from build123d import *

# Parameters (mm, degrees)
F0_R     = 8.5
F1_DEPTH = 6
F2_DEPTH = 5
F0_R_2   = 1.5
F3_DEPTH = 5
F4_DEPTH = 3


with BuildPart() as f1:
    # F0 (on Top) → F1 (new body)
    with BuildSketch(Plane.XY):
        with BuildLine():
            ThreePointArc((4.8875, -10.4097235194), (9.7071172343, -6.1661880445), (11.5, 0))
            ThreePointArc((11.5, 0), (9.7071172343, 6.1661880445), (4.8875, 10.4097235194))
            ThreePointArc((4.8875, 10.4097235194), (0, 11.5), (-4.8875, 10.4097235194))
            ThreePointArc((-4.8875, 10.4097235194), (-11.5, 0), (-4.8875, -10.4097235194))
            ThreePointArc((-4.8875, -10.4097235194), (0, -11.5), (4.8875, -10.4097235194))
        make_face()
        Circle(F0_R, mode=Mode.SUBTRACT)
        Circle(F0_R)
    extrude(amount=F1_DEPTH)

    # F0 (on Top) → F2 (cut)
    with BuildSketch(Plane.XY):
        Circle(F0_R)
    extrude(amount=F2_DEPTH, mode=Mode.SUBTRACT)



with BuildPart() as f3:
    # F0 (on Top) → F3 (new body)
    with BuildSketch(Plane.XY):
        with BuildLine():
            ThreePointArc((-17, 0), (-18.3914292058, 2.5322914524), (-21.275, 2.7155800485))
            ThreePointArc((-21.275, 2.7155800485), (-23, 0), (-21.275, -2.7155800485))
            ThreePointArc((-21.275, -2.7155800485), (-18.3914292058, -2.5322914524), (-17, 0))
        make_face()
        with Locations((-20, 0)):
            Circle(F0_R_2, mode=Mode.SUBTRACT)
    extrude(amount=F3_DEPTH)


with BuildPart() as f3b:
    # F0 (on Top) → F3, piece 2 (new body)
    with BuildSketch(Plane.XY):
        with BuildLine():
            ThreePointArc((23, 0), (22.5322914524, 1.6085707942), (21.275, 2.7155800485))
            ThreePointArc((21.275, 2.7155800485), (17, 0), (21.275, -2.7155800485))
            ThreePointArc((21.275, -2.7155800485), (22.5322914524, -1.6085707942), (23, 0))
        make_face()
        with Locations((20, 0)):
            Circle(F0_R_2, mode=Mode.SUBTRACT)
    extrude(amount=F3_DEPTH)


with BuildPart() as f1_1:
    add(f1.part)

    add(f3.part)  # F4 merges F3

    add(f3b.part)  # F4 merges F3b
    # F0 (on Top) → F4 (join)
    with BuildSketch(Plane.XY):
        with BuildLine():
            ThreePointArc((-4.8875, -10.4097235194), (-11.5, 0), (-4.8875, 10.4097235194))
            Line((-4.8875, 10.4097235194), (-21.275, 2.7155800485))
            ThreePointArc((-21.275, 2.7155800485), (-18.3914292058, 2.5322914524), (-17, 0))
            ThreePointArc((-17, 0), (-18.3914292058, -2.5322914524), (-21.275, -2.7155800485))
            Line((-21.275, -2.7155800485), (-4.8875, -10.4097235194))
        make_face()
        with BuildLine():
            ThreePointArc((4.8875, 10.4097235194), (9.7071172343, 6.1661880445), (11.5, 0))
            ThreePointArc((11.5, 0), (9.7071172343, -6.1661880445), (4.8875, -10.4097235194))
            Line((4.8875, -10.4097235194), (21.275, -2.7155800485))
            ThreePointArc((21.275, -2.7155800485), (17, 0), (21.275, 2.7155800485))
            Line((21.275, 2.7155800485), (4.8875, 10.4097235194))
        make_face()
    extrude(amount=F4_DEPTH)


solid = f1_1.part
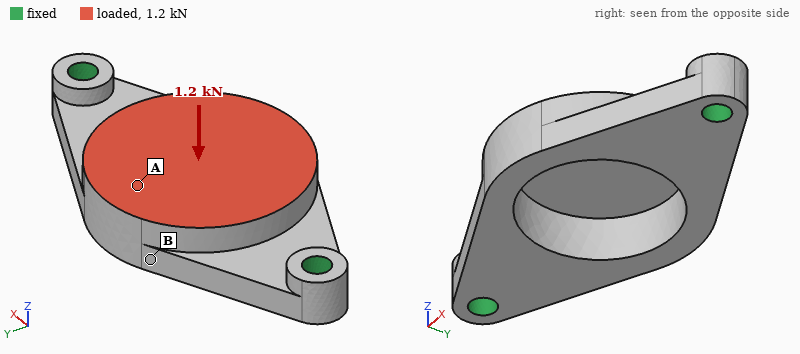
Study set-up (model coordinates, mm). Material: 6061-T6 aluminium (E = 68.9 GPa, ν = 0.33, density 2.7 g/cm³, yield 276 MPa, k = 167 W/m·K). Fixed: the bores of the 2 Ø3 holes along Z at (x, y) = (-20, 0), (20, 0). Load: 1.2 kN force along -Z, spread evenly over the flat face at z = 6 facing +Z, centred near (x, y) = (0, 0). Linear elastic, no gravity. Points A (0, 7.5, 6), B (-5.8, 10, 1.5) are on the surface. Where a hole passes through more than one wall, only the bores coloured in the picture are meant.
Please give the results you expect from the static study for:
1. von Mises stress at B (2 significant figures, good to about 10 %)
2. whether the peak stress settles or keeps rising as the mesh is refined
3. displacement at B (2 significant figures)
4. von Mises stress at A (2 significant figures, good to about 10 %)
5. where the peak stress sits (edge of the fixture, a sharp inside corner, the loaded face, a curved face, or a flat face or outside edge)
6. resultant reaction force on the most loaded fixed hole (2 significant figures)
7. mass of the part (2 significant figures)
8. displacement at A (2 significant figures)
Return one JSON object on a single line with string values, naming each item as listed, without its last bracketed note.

{"von Mises stress at B": "32 MPa", "whether the peak stress settles or keeps rising as the mesh is refined": "keeps rising", "displacement at B": "0.062 mm", "von Mises stress at A": "120 MPa", "where the peak stress sits": "edge of the fixture", "resultant reaction force on the most loaded fixed hole": "1.0 kN", "mass of the part": "5.8 g", "displacement at A": "0.069 mm"}
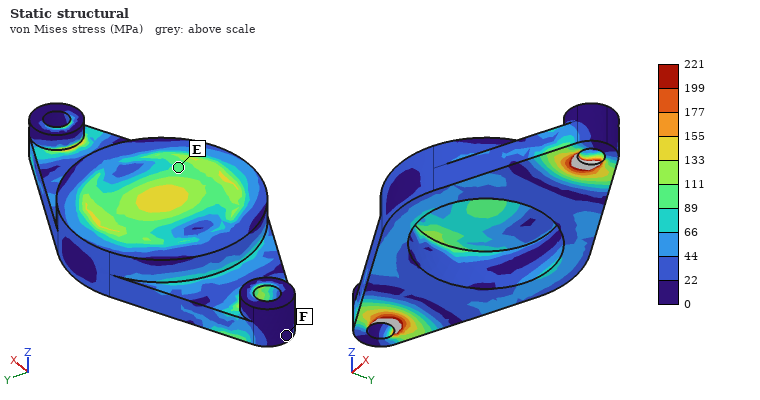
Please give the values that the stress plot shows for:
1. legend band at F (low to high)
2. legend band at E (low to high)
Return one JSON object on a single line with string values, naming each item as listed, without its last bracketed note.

{"legend band at F": "0 to 22 MPa", "legend band at E": "89 to 111 MPa"}
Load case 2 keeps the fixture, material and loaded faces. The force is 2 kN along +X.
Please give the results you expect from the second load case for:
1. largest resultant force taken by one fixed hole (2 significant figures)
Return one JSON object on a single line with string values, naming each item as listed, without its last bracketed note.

{"largest resultant force taken by one fixed hole": "1.0 kN"}
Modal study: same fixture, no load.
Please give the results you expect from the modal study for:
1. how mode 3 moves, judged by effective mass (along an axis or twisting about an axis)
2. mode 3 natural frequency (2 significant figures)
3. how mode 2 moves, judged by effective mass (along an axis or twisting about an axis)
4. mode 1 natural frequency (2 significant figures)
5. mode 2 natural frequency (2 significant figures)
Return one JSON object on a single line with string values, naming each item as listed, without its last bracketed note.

{"how mode 3 moves, judged by effective mass": "along Y", "mode 3 natural frequency": "23 kHz", "how mode 2 moves, judged by effective mass": "along Z", "mode 1 natural frequency": "8100 Hz", "mode 2 natural frequency": "11 kHz"}
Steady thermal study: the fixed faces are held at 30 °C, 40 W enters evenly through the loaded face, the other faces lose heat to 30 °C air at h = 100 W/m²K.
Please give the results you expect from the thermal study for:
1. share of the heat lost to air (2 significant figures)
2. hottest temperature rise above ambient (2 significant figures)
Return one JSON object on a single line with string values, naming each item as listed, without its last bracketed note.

{"share of the heat lost to air": "13 %", "hottest temperature rise above ambient": "51 K"}
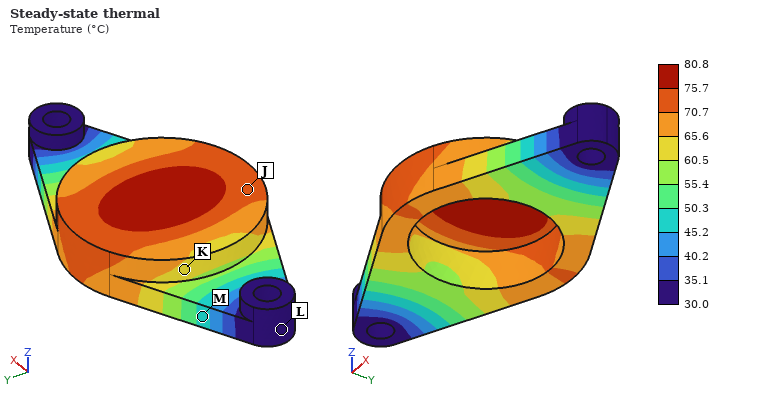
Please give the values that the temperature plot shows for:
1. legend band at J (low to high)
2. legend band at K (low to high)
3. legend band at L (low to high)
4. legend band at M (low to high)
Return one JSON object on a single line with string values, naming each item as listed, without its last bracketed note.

{"legend band at J": "70.7 to 75.7 °C", "legend band at K": "60.5 to 65.6 °C", "legend band at L": "30.0 to 35.1 °C", "legend band at M": "45.2 to 50.3 °C"}
